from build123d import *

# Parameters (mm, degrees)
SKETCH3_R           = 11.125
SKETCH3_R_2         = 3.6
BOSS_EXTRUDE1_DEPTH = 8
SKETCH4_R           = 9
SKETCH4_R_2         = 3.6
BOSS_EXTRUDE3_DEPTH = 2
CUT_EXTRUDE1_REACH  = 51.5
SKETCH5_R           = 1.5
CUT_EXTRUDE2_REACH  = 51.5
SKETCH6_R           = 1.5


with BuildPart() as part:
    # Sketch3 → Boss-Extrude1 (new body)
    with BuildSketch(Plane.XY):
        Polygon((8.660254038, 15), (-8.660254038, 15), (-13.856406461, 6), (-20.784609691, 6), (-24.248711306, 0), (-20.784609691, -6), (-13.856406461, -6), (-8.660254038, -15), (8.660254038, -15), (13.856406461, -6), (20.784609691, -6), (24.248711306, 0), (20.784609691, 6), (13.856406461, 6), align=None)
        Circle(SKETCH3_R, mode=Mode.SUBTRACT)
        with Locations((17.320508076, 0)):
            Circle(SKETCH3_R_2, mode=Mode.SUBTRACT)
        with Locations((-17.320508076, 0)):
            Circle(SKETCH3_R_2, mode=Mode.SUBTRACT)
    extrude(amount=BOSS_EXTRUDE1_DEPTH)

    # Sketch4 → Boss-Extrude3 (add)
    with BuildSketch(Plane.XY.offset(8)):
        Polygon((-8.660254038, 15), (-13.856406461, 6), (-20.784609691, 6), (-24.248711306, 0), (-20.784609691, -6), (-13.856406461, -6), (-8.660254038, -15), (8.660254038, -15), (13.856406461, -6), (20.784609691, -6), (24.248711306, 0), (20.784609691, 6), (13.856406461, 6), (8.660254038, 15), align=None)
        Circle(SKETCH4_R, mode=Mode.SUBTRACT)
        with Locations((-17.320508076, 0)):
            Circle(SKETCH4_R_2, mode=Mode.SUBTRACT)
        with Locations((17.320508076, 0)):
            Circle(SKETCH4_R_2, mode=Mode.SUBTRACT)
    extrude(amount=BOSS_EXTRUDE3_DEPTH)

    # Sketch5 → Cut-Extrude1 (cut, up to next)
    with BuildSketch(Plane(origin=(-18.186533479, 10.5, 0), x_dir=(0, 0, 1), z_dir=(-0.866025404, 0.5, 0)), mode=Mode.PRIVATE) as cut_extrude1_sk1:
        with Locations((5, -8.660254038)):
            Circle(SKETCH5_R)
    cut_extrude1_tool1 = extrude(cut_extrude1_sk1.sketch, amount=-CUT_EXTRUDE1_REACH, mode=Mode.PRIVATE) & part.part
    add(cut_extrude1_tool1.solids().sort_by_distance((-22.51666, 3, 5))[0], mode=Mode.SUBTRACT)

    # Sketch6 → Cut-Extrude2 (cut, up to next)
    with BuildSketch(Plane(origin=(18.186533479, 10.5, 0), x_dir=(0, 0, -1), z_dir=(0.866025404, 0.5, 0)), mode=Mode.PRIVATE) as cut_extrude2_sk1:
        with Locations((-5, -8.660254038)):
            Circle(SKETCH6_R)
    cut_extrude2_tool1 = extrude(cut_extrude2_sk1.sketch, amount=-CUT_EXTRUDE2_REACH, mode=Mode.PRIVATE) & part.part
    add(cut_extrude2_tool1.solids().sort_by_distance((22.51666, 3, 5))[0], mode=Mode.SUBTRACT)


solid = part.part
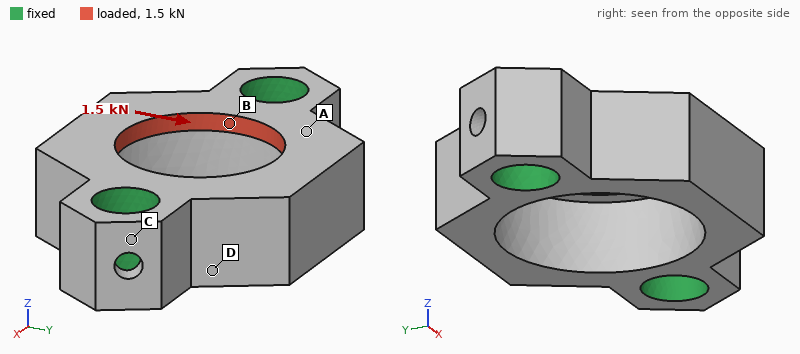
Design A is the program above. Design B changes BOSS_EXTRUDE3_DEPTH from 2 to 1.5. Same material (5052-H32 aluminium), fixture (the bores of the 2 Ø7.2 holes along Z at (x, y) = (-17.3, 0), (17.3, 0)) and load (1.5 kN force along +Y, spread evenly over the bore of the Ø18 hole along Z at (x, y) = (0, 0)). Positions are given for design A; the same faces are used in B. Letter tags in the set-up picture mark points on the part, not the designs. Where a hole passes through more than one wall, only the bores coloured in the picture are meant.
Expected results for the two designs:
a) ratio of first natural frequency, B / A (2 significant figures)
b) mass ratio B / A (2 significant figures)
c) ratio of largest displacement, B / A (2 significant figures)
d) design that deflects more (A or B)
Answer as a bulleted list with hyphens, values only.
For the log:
- 0.97
- 0.94
- 1.1
- B
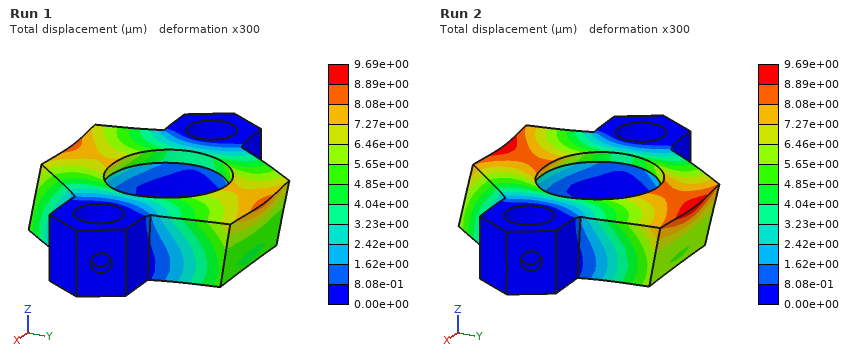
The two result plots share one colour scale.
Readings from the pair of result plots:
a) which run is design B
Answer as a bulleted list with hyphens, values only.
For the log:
- Run 2
